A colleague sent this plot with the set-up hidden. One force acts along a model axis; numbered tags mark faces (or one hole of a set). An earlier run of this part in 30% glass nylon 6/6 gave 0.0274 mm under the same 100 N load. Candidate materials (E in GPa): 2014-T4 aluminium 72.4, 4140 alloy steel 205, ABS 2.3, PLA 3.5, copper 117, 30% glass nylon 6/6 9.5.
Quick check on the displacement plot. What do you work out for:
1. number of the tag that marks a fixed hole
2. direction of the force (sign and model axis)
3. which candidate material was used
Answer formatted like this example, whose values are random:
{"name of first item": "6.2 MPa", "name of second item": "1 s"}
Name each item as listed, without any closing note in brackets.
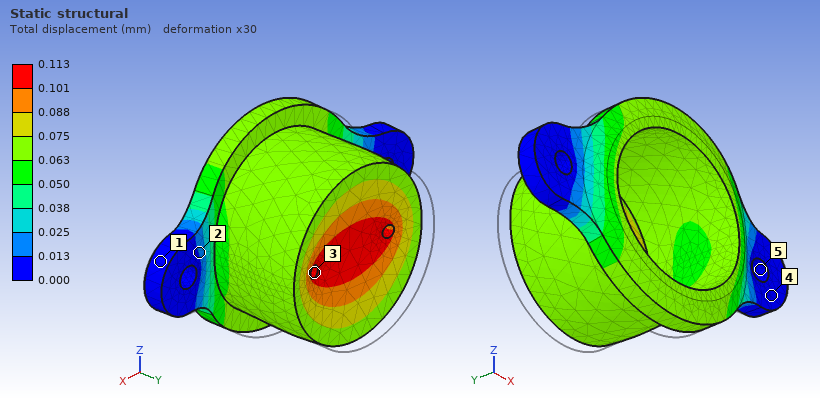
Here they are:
{"number of the tag that marks a fixed hole": "5", "direction of the force": "-Y", "which candidate material was used": "ABS"}
